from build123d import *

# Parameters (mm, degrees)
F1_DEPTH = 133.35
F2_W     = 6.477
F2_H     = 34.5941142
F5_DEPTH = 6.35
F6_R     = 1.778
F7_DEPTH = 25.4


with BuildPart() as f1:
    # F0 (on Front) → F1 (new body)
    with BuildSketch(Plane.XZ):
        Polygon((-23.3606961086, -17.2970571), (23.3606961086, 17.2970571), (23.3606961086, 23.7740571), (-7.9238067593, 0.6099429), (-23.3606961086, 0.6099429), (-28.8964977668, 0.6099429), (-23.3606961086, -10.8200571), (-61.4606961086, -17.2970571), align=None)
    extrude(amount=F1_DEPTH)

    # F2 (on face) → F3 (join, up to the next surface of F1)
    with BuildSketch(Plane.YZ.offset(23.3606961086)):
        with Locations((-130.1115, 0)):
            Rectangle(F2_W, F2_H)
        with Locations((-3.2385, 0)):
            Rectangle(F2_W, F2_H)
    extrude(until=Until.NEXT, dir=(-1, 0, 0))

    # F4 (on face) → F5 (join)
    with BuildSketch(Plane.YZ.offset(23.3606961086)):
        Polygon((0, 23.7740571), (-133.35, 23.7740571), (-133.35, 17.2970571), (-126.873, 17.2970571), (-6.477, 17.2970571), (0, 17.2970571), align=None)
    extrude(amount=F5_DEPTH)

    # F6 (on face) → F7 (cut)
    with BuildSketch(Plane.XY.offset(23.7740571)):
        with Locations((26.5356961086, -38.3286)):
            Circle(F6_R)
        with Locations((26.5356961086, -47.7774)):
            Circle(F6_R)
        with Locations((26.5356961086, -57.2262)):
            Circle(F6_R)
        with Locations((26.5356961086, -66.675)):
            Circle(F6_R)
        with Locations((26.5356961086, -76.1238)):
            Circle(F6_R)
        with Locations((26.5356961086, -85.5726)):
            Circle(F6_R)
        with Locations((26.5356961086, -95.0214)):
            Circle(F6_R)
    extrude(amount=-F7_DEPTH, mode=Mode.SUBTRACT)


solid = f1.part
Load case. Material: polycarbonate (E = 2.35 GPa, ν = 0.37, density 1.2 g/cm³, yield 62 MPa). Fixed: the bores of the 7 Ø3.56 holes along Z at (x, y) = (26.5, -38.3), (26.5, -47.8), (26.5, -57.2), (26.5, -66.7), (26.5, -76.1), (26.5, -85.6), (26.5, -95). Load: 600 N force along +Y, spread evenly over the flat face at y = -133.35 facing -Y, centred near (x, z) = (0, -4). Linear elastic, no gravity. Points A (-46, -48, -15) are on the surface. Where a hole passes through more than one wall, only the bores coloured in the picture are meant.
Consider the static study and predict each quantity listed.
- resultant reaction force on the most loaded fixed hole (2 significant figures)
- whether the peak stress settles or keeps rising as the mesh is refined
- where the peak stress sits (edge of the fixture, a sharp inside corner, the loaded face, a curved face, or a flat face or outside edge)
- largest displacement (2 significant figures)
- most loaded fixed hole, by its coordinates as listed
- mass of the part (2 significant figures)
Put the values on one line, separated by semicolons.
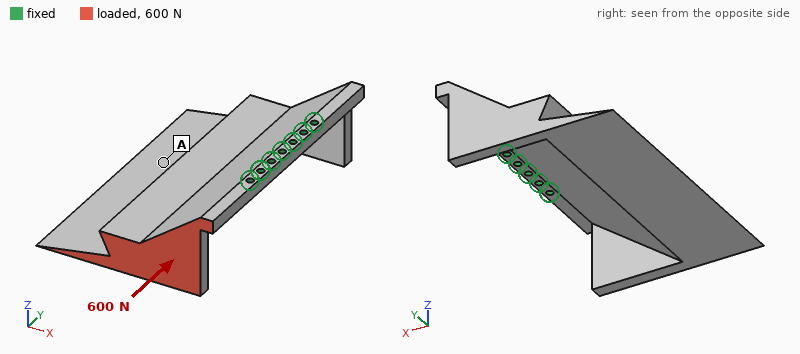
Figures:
330 N; keeps rising; edge of the fixture; 1.9 mm; (26.5, -95); 110 g
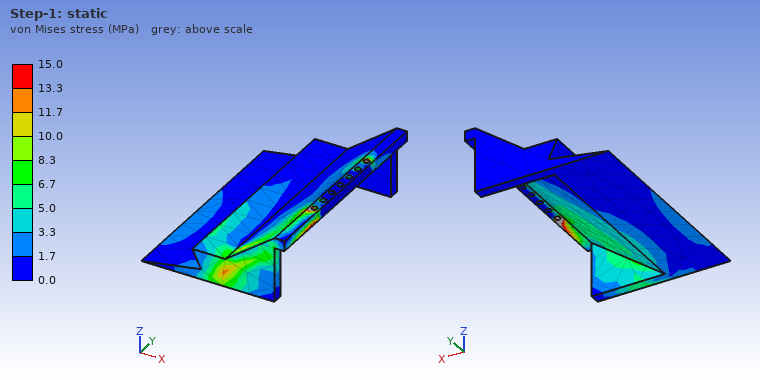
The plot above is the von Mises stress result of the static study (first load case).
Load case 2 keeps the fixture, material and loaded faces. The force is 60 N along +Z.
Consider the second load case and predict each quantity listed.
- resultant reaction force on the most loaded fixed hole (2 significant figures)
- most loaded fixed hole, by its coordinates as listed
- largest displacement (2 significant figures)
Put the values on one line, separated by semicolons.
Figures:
76 N; (26.5, -95); 1.5 mm
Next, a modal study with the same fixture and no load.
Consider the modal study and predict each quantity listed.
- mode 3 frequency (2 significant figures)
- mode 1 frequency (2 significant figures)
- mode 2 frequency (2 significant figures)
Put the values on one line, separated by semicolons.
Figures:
650 Hz; 150 Hz; 230 Hz
